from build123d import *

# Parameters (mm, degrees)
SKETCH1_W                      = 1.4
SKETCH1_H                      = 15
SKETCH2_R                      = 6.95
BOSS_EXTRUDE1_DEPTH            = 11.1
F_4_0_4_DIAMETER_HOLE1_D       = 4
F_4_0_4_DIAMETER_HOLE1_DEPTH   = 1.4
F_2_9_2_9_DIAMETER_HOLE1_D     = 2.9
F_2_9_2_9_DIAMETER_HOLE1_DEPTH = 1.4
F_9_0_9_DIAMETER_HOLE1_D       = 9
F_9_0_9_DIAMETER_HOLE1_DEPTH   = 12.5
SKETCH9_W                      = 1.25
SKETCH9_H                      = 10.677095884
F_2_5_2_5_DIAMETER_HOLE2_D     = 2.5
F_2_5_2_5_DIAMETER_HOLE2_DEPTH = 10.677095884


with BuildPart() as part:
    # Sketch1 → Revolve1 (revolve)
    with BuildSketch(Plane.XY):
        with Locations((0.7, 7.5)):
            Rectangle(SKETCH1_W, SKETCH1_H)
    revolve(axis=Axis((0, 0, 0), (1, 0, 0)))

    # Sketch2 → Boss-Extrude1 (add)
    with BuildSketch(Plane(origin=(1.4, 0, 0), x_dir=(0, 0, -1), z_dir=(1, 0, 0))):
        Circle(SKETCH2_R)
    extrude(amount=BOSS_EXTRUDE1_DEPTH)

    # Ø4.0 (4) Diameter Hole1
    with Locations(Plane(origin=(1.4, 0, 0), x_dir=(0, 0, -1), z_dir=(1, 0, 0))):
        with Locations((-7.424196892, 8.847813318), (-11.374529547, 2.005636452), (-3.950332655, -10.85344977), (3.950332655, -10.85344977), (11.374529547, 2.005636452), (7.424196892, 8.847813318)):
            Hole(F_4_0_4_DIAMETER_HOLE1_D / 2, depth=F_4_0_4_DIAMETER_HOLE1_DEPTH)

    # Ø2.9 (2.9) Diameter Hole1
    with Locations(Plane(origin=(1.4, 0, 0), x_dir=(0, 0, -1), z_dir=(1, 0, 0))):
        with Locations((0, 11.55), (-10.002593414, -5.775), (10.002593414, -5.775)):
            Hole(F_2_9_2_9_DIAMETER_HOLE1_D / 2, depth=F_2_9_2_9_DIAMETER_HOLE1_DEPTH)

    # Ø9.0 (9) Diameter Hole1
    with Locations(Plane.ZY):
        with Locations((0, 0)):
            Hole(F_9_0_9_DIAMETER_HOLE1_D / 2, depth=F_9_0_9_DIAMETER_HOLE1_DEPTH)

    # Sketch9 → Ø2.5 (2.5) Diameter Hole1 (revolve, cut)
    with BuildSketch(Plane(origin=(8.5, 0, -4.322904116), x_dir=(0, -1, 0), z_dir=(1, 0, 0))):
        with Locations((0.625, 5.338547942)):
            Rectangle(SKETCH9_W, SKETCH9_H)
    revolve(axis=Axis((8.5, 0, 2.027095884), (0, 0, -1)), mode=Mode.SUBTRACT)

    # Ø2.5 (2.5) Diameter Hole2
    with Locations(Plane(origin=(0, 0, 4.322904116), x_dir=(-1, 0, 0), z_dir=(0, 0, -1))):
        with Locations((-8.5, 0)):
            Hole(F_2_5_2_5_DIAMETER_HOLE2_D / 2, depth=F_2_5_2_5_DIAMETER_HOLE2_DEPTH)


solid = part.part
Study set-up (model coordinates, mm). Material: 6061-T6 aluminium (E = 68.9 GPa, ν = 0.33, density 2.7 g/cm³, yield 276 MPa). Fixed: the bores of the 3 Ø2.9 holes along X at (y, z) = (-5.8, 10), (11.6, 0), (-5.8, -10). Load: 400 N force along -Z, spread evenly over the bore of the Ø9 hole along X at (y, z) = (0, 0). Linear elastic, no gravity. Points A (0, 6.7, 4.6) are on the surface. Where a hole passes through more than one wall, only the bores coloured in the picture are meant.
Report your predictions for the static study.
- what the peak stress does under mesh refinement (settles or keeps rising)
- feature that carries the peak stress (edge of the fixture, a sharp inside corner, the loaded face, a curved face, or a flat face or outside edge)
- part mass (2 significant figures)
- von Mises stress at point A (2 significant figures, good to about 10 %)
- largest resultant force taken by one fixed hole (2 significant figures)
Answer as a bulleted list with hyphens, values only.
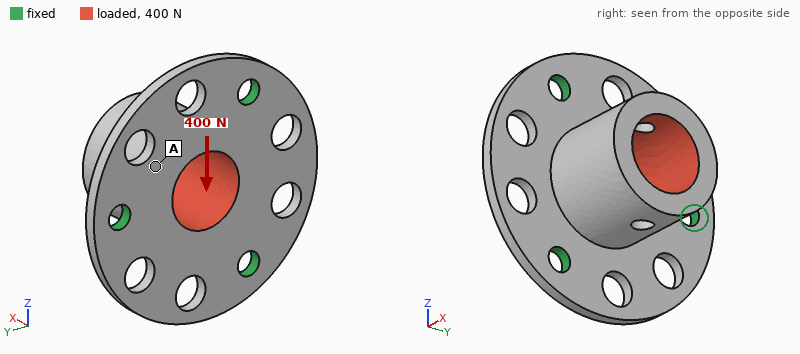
- keeps rising
- edge of the fixture
- 4.6 g
- 12 MPa
- 200 N
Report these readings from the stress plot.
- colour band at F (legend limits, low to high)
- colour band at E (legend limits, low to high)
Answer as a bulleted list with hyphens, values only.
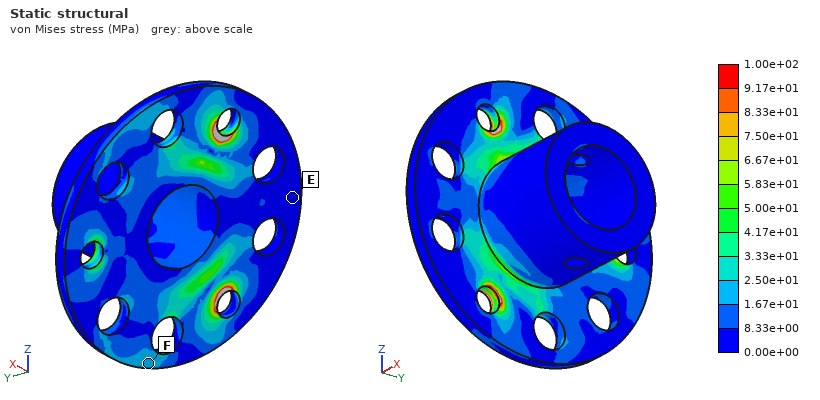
- 1.67e+01 to 2.50e+01 MPa
- 0.00e+00 to 8.33e+00 MPa
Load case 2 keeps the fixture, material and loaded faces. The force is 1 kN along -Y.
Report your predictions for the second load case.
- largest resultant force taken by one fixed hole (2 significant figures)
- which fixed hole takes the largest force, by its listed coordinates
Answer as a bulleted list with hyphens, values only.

- 560 N
- (11.6, 0)
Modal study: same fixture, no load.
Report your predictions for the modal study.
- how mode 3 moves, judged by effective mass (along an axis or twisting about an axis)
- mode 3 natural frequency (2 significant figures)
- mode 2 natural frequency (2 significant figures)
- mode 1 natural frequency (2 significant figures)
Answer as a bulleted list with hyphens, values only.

- along X
- 15 kHz
- 13 kHz
- 13 kHz
